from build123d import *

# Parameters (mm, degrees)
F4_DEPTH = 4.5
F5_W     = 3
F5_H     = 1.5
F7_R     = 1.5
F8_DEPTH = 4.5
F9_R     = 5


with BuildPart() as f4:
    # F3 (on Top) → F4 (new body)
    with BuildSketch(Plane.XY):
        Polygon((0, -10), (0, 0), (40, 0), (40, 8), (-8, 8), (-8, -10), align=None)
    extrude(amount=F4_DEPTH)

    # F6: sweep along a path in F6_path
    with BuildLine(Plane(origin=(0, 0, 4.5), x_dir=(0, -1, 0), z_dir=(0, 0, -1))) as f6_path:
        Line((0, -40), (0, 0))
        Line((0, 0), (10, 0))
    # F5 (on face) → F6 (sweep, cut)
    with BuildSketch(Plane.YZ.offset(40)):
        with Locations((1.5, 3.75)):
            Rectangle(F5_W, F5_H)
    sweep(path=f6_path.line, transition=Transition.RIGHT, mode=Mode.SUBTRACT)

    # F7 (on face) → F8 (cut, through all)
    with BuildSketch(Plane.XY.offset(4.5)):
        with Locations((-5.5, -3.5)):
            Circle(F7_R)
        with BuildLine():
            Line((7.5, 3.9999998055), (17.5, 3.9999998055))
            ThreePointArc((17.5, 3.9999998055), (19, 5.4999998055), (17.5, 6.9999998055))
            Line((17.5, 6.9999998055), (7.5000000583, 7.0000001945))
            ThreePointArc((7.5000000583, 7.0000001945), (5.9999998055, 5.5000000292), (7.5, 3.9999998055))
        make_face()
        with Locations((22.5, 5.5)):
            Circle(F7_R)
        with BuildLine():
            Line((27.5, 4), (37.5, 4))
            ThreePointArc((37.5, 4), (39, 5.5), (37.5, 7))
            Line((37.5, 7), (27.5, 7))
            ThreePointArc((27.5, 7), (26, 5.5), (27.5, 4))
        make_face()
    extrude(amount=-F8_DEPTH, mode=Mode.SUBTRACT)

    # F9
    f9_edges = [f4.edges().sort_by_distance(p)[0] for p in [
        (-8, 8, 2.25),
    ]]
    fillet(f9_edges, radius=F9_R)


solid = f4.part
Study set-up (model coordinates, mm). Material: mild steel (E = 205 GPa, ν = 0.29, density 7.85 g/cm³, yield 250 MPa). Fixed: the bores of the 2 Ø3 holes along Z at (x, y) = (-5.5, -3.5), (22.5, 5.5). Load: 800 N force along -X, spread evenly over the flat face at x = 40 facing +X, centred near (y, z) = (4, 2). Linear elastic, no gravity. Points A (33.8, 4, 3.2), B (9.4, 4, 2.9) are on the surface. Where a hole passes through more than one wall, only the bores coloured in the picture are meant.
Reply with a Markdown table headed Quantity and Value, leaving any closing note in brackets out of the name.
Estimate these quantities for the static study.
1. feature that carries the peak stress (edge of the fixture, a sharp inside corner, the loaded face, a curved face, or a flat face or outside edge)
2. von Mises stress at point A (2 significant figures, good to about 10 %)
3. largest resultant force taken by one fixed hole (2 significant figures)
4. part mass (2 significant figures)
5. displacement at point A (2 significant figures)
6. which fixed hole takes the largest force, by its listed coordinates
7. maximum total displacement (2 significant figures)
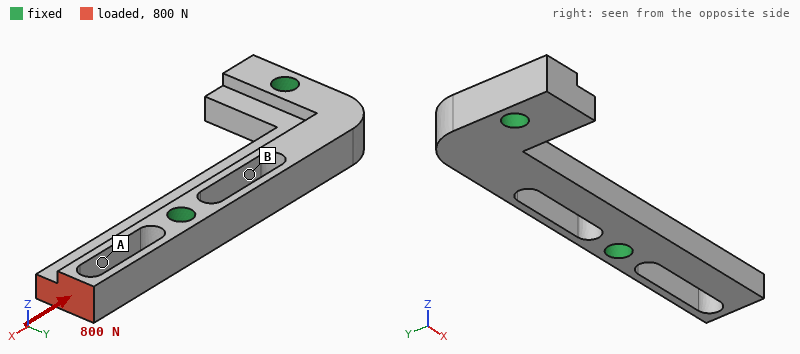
| Quantity | Value |
|---|---|
| feature that carries the peak stress | a curved face |
| von Mises stress at point A | 73 MPa |
| largest resultant force taken by one fixed hole | 780 N |
| part mass | 11 g |
| displacement at point A | 3.2 µm |
| which fixed hole takes the largest force, by its listed coordinates | (22.5, 5.5) |
| maximum total displacement | 8.8 µm |
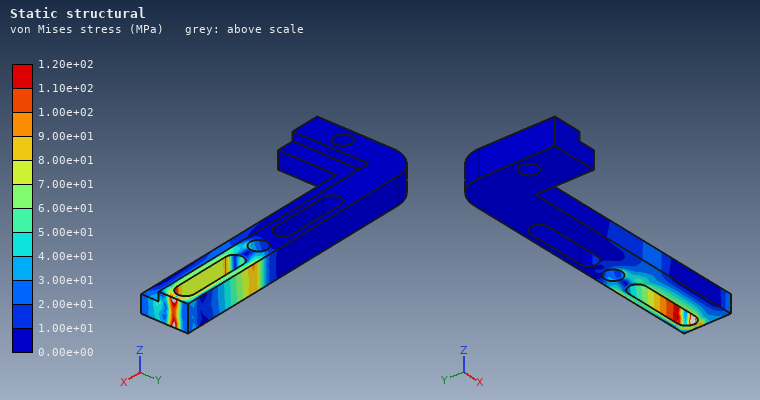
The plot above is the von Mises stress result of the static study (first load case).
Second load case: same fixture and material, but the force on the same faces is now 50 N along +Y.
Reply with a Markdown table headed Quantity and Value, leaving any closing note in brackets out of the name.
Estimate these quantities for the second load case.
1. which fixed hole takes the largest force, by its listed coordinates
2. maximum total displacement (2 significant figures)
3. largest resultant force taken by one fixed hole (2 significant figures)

| Quantity | Value |
|---|---|
| which fixed hole takes the largest force, by its listed coordinates | (22.5, 5.5) |
| maximum total displacement | 12 µm |
| largest resultant force taken by one fixed hole | 58 N |
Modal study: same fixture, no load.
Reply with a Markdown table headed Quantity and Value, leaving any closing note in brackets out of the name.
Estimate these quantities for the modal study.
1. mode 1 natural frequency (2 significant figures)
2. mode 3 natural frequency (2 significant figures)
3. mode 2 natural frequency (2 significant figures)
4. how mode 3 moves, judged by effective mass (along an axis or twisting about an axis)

| Quantity | Value |
|---|---|
| mode 1 natural frequency | 10 kHz |
| mode 3 natural frequency | 19 kHz |
| mode 2 natural frequency | 12 kHz |
| how mode 3 moves, judged by effective mass | along Z |
